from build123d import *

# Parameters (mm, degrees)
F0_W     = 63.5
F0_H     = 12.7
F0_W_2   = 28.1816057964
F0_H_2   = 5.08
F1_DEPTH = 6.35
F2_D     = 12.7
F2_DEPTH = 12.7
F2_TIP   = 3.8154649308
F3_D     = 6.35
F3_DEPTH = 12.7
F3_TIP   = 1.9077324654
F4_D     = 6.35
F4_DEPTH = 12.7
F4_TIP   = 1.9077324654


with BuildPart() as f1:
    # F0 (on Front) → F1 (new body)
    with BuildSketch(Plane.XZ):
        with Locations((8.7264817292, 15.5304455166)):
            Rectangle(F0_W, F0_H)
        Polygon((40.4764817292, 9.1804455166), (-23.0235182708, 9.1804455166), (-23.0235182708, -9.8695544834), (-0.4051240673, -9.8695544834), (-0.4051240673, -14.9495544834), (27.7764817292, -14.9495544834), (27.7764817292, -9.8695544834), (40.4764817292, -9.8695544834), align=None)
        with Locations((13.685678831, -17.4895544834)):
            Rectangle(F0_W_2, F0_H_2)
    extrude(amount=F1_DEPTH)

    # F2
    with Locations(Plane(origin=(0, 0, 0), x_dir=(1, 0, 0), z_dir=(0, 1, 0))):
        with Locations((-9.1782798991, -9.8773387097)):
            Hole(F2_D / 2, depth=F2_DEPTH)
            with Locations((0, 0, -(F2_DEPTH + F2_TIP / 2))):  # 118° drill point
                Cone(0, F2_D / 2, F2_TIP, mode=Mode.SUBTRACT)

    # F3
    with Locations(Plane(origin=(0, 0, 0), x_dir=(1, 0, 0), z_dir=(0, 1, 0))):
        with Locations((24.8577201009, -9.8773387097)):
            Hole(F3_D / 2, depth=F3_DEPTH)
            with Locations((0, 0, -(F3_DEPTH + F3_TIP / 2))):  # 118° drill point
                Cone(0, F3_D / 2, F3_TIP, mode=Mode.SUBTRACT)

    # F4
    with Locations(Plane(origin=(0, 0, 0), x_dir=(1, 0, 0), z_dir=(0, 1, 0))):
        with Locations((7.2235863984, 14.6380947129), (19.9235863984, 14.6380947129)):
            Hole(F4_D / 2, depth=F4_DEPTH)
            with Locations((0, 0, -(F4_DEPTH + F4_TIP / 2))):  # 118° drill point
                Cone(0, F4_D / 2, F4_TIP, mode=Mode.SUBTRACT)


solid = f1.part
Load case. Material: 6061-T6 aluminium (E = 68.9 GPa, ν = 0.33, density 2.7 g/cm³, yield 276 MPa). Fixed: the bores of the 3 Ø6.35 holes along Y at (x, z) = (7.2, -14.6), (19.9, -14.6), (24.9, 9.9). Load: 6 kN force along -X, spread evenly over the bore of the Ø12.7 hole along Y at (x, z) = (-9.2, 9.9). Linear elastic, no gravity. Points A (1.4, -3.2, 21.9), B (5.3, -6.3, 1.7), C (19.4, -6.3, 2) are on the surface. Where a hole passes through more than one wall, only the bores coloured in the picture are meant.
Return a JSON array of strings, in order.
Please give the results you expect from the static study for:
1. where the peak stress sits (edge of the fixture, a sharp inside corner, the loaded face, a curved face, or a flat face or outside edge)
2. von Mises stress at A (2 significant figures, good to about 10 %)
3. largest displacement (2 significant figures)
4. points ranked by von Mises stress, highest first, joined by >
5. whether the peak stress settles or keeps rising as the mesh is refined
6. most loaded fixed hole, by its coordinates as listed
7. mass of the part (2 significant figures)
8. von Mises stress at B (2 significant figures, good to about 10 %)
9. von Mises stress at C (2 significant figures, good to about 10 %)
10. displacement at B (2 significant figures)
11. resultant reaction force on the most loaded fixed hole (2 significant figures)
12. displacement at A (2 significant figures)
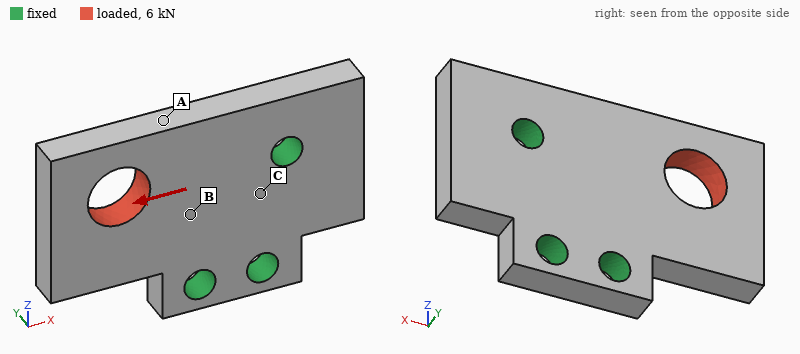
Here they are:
["edge of the fixture", "64 MPa", "40 µm", "A > B > C", "keeps rising", "(24.9, 9.9)", "36 g", "33 MPa", "14 MPa", "7.7 µm", "5.1 kN", "24 µm"]
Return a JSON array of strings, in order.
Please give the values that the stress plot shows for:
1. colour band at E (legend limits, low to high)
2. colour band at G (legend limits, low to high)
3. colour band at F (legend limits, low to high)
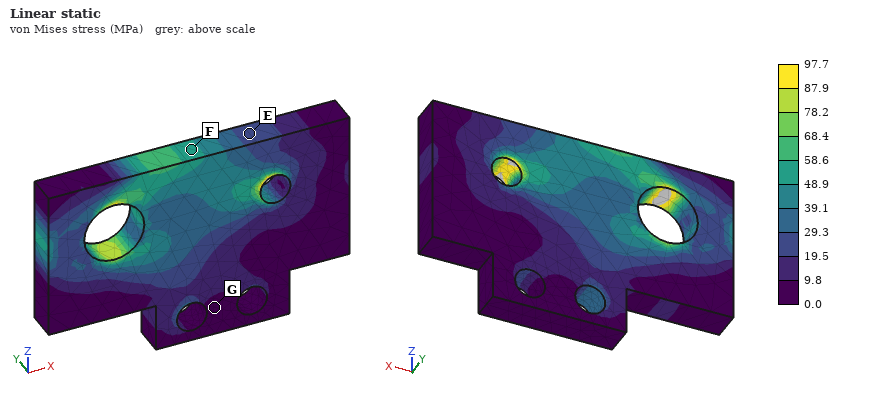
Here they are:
["19.5 to 29.3 MPa", "0.0 to 9.8 MPa", "48.9 to 58.6 MPa"]
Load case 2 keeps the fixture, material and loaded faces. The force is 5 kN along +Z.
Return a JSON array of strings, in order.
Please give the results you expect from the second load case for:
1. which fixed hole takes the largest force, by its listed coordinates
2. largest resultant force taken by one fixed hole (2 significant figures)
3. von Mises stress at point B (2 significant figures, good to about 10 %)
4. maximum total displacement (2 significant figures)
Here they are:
["(7.2, -14.6)", "5.0 kN", "50 MPa", "70 µm"]
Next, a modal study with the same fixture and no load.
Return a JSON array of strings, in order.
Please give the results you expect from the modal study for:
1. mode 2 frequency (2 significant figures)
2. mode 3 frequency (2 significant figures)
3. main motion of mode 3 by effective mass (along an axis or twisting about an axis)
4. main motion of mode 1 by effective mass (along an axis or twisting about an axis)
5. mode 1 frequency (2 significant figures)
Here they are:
["8800 Hz", "13 kHz", "along Z", "along Y", "3700 Hz"]
